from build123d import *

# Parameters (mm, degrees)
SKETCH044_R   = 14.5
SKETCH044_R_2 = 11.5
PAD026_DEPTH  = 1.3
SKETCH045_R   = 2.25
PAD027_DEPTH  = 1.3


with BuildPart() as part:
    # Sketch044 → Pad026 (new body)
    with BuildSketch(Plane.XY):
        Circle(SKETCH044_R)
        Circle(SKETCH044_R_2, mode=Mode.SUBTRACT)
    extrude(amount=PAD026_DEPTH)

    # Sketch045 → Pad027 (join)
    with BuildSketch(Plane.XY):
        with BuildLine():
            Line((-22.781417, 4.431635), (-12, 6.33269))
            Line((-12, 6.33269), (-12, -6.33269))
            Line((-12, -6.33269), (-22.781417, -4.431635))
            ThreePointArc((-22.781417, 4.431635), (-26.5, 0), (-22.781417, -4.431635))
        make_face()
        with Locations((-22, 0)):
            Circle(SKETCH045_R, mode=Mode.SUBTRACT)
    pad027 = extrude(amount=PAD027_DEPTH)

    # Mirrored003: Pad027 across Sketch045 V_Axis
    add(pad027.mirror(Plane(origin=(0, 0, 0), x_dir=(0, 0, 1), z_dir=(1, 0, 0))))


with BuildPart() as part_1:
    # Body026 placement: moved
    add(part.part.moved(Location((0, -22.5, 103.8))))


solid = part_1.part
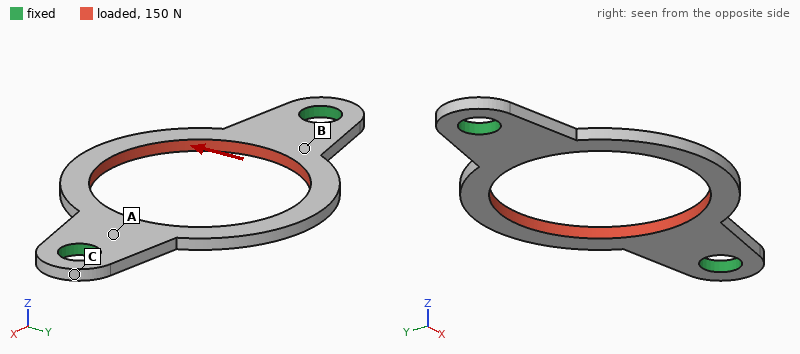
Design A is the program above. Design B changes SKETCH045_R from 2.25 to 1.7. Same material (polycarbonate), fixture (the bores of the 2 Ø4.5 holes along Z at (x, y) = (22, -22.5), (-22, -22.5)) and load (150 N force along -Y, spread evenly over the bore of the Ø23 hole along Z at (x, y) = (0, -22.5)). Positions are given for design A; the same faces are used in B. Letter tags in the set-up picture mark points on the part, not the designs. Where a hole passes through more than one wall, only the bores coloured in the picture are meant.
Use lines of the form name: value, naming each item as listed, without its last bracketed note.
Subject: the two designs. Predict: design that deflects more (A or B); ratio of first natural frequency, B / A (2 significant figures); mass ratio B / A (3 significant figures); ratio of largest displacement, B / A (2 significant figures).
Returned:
design that deflects more: B
ratio of first natural frequency, B / A: 0.96
mass ratio B / A: 1.03
ratio of largest displacement, B / A: 1.3
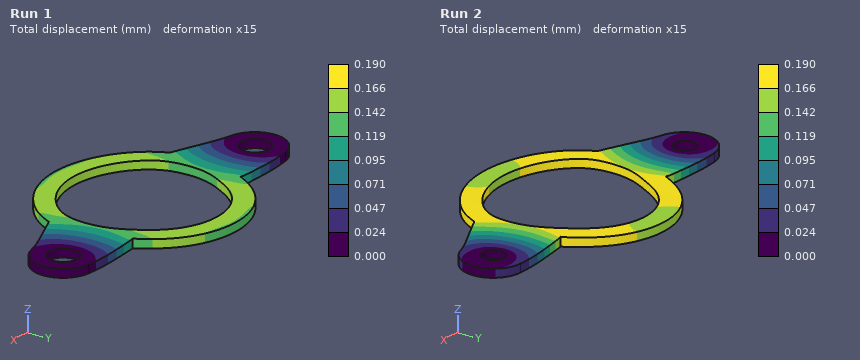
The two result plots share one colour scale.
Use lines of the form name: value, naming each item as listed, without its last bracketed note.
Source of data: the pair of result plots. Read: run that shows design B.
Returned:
run that shows design B: Run 2
